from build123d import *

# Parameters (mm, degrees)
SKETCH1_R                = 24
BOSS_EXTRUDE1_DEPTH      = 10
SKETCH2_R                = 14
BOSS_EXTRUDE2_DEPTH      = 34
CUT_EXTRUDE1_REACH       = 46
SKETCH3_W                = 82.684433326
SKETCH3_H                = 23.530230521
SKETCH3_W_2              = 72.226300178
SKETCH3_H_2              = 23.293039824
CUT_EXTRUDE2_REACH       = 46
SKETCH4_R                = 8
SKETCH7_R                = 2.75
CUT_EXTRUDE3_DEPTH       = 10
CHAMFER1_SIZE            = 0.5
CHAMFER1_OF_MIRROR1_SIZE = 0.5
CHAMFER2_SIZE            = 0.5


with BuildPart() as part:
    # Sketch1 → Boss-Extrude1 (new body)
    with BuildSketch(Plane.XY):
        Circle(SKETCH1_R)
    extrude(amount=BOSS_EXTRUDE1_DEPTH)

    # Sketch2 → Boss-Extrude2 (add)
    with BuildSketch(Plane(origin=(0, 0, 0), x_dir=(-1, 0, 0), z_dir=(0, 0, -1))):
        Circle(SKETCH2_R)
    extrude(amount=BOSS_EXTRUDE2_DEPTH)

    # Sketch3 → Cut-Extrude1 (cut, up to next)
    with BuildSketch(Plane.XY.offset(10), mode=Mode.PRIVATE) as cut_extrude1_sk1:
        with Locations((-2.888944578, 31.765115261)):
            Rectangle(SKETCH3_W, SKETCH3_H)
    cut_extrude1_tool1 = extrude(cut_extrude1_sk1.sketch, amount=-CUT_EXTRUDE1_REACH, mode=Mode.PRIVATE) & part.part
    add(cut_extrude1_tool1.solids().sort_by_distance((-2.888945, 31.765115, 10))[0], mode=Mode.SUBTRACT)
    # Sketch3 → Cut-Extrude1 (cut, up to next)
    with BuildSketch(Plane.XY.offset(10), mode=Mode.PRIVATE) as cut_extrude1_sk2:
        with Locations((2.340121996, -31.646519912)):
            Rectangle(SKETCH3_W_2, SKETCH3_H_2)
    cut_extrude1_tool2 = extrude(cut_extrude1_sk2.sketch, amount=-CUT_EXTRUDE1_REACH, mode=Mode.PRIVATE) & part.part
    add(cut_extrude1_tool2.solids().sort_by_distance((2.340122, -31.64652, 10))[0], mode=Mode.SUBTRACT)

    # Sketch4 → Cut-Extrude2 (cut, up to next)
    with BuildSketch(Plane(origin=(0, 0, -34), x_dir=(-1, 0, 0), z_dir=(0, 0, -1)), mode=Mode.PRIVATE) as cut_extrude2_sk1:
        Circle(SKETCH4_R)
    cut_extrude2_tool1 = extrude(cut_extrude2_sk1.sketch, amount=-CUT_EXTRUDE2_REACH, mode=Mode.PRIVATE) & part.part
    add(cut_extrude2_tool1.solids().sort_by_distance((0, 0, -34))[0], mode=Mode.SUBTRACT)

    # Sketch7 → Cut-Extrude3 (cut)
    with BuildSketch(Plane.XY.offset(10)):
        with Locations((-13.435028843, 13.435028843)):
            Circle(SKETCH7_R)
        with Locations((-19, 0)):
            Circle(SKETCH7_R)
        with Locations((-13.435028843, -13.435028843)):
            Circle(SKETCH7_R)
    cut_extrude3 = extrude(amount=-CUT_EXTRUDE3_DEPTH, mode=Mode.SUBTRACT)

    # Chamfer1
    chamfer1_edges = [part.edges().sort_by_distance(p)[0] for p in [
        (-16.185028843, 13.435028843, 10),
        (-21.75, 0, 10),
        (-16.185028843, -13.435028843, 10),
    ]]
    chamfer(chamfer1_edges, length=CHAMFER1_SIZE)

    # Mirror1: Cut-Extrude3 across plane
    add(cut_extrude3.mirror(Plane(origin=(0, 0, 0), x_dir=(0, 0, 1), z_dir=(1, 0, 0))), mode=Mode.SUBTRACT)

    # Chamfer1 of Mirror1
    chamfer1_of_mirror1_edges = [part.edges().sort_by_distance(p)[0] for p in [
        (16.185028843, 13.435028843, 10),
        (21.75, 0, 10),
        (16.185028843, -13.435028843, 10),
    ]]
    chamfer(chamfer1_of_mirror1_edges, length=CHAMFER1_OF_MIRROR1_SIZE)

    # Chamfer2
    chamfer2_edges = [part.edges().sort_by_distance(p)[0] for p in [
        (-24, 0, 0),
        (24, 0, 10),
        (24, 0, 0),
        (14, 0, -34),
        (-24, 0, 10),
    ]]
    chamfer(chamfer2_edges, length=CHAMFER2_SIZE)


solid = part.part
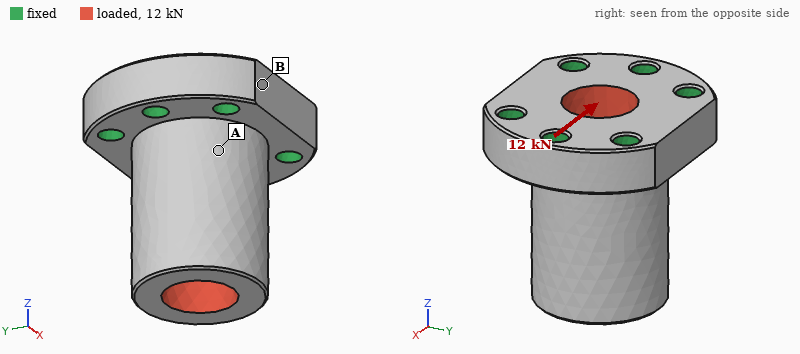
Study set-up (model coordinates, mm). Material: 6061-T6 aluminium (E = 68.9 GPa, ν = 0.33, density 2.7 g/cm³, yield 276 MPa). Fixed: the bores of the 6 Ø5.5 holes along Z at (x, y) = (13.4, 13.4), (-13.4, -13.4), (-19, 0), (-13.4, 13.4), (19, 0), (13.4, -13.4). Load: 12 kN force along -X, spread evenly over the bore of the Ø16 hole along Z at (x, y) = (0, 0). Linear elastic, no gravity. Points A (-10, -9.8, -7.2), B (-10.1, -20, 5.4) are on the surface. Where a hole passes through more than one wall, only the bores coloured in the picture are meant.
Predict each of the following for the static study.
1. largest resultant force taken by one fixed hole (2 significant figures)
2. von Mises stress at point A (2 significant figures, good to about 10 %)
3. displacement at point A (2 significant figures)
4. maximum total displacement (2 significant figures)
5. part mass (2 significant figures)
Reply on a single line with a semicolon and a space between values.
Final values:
3.9 kN; 42 MPa; 20 µm; 72 µm; 74 g
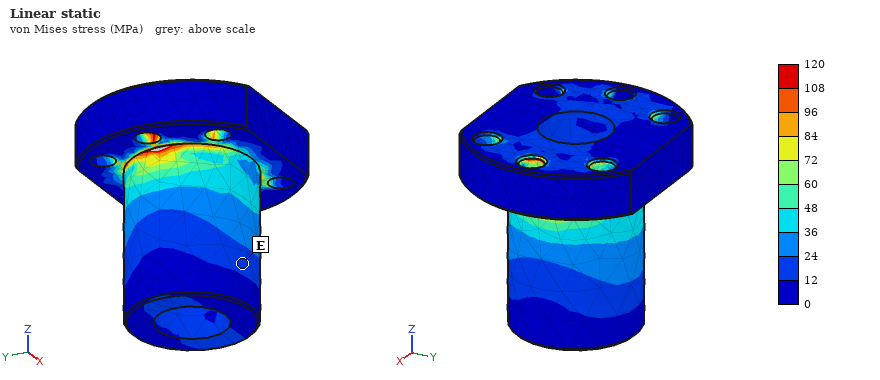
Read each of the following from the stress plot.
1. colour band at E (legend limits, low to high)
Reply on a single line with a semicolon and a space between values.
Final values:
12 to 24 MPa
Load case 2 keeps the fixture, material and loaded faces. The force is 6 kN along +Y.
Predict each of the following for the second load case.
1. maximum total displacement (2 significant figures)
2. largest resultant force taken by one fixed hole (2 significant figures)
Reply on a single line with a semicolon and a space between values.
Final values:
43 µm; 2.3 kN
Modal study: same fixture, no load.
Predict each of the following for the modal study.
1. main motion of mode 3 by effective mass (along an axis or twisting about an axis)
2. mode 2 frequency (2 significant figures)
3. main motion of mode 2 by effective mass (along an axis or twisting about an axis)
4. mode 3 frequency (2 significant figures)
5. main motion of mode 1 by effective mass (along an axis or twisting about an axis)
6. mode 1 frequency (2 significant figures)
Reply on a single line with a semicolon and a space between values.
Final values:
twisting about Z; 11 kHz; along X; 21 kHz; along Y; 10 kHz
